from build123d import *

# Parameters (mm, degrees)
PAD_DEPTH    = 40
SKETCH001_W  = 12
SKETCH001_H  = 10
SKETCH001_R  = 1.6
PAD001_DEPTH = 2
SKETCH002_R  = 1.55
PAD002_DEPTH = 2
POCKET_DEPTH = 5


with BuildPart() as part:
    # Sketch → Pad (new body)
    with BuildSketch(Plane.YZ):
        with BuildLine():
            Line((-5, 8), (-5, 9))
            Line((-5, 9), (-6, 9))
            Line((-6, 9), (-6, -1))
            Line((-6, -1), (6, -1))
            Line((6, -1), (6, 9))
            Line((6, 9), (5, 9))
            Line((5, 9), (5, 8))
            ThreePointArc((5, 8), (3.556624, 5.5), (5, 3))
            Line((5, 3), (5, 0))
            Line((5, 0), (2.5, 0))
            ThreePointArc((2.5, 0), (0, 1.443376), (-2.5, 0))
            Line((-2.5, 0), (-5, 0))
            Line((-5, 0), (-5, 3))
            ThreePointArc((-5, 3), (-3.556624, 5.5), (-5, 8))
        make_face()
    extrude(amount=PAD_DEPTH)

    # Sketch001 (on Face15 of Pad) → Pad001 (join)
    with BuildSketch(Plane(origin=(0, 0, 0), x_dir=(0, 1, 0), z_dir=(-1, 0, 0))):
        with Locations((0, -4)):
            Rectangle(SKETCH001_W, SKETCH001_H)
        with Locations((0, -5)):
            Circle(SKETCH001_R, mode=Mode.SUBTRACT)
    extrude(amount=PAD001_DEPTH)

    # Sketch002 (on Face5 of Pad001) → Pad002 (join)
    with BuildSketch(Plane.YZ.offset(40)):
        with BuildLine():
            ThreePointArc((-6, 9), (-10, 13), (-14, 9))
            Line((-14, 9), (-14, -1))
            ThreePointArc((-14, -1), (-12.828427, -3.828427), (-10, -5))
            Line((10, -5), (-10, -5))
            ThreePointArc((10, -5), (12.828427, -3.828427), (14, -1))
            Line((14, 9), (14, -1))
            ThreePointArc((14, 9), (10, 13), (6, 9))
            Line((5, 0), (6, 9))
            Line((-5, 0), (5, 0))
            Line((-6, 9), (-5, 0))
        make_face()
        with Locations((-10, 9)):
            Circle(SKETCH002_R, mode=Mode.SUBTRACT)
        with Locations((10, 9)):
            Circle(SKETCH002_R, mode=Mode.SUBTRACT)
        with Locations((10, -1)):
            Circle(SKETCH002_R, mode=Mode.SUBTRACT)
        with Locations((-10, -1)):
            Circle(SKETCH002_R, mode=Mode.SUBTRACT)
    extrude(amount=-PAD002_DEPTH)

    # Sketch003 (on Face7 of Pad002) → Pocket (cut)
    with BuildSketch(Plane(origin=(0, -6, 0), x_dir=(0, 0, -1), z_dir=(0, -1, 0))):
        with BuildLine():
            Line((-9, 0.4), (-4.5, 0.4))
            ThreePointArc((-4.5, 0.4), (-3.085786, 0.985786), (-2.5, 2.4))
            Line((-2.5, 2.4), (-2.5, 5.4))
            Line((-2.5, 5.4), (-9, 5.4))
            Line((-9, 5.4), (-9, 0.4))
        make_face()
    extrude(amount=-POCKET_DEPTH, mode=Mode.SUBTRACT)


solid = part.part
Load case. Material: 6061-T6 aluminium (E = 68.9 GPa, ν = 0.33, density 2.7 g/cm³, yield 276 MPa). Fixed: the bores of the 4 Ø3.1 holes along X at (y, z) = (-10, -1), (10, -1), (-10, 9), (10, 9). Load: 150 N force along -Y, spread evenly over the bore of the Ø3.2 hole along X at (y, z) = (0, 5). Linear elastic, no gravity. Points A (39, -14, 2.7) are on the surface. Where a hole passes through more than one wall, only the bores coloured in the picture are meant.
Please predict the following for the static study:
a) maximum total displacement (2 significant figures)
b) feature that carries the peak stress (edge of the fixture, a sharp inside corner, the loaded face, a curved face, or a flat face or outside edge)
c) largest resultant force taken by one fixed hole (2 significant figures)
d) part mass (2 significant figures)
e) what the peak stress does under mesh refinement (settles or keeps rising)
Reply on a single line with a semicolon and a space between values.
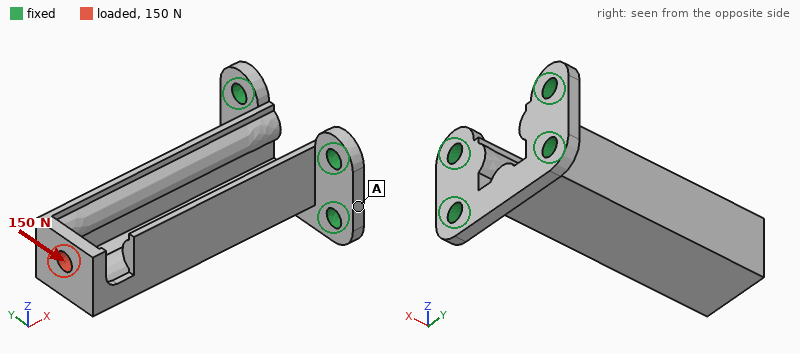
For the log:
0.48 mm; a sharp inside corner; 360 N; 6.9 g; keeps rising
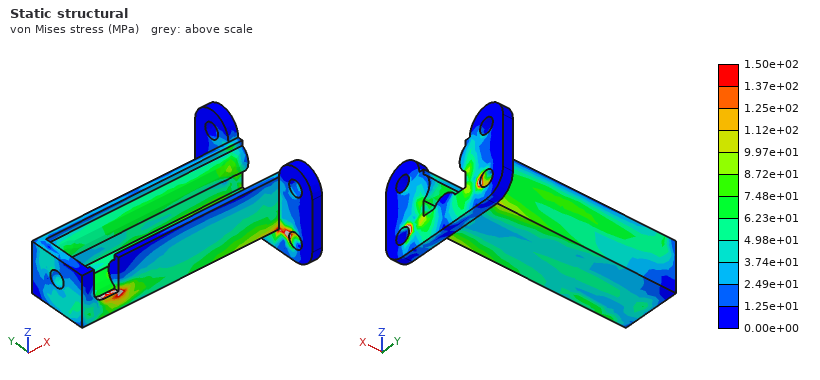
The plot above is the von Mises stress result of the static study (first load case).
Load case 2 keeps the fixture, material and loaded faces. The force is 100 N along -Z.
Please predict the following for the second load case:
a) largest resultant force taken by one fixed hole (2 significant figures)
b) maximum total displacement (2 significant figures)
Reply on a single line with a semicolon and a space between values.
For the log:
220 N; 0.20 mm
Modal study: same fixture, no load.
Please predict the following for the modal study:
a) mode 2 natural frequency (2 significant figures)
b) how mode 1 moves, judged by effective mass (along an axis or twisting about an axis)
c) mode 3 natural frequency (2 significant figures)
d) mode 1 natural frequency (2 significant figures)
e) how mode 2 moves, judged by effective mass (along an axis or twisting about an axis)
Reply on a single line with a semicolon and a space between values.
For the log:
2800 Hz; along Y; 6400 Hz; 2600 Hz; along Z
